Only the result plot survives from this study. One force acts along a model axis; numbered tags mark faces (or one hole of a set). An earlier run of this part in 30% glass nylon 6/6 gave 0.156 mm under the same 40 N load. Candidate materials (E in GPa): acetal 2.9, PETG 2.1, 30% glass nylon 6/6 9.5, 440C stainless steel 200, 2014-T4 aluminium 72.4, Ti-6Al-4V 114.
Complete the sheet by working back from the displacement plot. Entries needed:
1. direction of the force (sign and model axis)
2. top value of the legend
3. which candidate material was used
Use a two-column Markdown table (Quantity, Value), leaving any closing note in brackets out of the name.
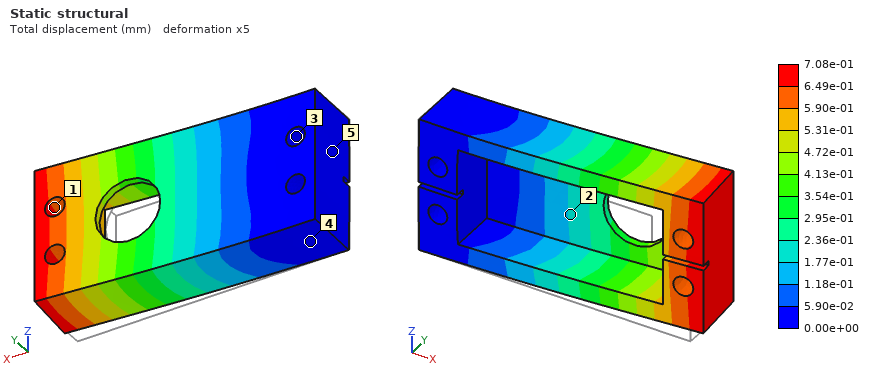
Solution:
| Quantity | Value |
|---|---|
| direction of the force | +Y |
| top value of the legend | 7.08e-01 mm |
| which candidate material was used | PETG |
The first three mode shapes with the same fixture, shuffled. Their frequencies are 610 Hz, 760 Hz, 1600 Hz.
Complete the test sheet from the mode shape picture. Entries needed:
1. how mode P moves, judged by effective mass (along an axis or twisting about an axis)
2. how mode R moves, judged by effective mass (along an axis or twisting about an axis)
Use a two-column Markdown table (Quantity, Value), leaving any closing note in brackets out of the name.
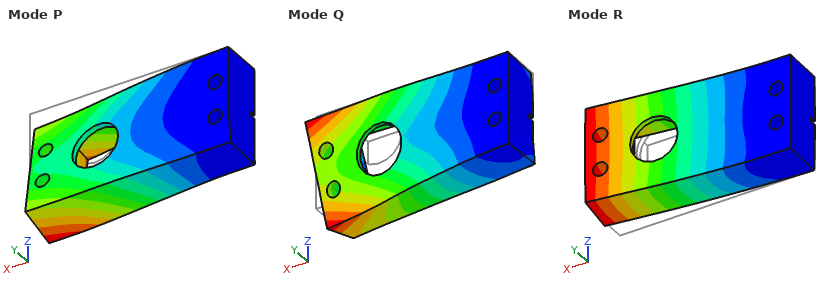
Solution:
| Quantity | Value |
|---|---|
| how mode P moves, judged by effective mass | along Z |
| how mode R moves, judged by effective mass | along Y |
